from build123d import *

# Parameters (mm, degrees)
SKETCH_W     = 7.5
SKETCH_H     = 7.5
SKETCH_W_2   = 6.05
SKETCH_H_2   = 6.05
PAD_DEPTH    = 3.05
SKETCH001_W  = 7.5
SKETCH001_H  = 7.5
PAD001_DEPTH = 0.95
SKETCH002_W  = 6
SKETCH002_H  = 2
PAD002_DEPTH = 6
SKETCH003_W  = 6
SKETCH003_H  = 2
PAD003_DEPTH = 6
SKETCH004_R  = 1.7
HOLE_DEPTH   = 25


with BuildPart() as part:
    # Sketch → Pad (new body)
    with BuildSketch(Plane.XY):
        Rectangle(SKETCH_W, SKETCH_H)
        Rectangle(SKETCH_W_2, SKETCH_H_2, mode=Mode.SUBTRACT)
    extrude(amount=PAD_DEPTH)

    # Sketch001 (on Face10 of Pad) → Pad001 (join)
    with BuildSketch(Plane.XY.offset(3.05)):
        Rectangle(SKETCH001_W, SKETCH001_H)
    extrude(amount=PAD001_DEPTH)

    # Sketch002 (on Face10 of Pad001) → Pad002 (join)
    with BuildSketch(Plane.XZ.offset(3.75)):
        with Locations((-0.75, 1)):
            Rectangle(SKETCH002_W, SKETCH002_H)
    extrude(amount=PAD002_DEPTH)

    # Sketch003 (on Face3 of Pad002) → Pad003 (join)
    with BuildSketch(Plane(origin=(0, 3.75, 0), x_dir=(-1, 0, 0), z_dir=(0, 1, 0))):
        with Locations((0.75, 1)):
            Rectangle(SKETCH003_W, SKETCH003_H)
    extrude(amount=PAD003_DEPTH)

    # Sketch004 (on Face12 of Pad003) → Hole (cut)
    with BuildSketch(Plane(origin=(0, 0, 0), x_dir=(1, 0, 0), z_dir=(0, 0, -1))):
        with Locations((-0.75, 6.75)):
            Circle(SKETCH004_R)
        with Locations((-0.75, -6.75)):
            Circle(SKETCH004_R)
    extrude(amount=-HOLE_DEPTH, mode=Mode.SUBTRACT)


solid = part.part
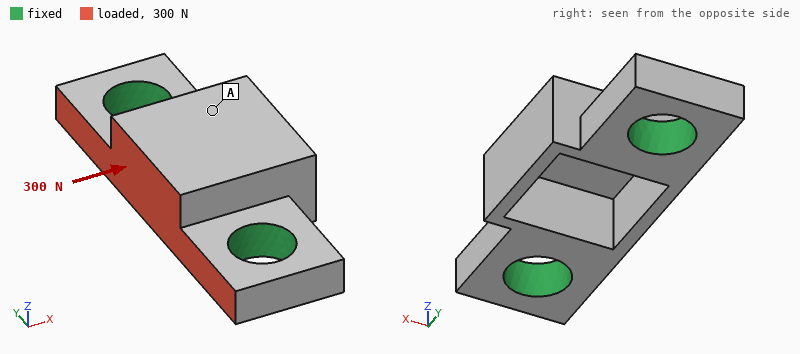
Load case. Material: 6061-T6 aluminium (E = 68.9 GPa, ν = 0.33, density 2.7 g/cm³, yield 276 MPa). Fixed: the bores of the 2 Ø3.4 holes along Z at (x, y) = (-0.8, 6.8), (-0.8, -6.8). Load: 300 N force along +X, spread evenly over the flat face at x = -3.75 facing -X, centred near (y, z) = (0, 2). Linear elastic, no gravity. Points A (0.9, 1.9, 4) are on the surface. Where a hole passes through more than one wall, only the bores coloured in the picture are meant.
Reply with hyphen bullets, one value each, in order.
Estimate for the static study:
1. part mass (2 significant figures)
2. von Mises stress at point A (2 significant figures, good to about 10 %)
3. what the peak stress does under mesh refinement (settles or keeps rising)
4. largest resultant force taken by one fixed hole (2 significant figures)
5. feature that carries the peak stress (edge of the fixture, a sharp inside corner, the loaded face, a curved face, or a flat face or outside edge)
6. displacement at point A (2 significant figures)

- 0.60 g
- 12 MPa
- keeps rising
- 150 N
- a sharp inside corner
- 3.1 µm
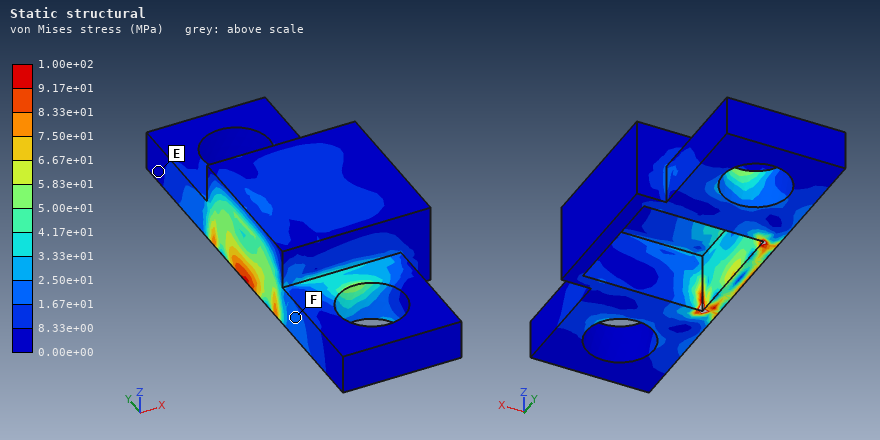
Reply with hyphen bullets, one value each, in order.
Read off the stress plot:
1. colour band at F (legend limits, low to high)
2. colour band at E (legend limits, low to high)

- 1.67e+01 to 2.50e+01 MPa
- 0.00e+00 to 8.33e+00 MPa
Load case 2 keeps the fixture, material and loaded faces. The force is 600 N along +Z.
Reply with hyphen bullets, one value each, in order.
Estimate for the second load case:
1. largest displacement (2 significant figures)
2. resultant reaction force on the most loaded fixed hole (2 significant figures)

- 24 µm
- 310 N
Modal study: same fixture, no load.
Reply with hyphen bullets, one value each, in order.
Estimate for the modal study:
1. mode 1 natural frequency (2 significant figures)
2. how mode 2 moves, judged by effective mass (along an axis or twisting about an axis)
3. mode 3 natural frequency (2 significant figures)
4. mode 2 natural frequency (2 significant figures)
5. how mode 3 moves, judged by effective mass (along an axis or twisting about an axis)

- 50 kHz
- along Y
- 80 kHz
- 76 kHz
- along Z
